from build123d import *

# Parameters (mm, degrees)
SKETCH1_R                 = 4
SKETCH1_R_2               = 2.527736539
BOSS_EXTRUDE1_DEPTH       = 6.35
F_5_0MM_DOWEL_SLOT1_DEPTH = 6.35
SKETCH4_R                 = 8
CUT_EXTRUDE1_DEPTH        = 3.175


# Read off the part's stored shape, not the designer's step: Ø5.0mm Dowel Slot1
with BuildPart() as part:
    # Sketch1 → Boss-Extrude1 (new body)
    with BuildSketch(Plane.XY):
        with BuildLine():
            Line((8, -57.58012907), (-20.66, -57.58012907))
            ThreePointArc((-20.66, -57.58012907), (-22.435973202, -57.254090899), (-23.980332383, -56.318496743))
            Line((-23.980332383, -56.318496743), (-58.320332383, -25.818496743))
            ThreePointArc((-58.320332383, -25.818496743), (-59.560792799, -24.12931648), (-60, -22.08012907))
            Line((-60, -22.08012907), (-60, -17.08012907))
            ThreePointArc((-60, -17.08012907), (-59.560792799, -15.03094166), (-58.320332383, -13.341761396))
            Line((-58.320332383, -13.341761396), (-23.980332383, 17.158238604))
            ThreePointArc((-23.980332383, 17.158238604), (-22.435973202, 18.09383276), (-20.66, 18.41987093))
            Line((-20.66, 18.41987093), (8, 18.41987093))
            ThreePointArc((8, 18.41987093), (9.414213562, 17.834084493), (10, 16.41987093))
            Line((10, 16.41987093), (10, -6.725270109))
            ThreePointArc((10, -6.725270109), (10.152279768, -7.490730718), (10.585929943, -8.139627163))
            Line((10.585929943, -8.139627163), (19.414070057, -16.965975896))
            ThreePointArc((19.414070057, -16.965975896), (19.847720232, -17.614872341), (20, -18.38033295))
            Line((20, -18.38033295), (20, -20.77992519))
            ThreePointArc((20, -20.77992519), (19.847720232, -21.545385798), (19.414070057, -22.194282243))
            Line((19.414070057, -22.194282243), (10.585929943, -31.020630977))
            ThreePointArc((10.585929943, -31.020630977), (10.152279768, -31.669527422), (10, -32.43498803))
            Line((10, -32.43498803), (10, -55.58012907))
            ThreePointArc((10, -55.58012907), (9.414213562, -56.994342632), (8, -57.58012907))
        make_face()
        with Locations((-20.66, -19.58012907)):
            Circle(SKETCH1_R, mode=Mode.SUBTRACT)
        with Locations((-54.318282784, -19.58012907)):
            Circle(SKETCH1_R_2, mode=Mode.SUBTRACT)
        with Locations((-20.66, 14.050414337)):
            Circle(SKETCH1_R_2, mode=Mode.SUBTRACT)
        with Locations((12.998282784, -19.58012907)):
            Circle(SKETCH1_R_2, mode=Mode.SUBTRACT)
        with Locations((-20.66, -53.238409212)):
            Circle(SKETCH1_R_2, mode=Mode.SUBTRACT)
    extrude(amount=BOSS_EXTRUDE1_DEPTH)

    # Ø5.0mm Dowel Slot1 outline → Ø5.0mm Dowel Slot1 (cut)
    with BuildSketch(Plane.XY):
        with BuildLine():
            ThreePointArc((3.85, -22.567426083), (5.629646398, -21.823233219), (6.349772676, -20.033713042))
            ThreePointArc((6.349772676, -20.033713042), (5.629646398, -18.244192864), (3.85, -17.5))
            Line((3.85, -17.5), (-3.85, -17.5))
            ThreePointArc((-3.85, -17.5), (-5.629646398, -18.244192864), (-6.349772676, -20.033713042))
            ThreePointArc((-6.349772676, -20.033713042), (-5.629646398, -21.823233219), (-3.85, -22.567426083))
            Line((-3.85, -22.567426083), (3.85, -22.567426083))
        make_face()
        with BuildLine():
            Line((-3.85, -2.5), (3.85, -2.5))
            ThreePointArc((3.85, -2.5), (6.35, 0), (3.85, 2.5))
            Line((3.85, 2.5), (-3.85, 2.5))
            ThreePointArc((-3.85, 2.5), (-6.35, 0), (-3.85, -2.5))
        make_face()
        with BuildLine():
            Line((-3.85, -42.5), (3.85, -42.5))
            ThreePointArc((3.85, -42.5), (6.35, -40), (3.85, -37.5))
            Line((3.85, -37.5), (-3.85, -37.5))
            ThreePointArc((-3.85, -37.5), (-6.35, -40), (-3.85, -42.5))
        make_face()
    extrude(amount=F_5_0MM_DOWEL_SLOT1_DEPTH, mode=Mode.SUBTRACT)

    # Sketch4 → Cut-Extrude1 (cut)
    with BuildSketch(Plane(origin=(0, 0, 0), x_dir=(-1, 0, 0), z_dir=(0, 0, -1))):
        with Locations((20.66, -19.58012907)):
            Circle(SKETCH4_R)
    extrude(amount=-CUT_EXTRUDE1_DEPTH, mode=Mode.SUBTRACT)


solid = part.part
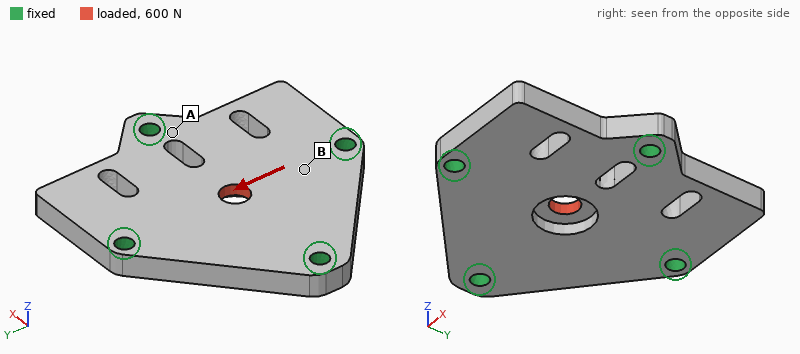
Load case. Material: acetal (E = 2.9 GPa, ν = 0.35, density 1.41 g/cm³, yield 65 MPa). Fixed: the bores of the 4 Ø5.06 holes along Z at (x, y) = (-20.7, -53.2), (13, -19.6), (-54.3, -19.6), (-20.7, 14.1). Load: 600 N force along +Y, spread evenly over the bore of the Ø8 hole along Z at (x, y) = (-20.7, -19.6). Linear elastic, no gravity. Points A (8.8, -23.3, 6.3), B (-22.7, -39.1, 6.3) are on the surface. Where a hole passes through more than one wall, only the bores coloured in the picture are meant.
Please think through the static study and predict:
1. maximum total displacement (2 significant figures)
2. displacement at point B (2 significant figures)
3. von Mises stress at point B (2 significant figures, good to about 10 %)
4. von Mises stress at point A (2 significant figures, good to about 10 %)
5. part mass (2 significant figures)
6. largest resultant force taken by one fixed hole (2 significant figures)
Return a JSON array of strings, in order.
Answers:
["38 µm", "12 µm", "3.0 MPa", "1.2 MPa", "34 g", "230 N"]
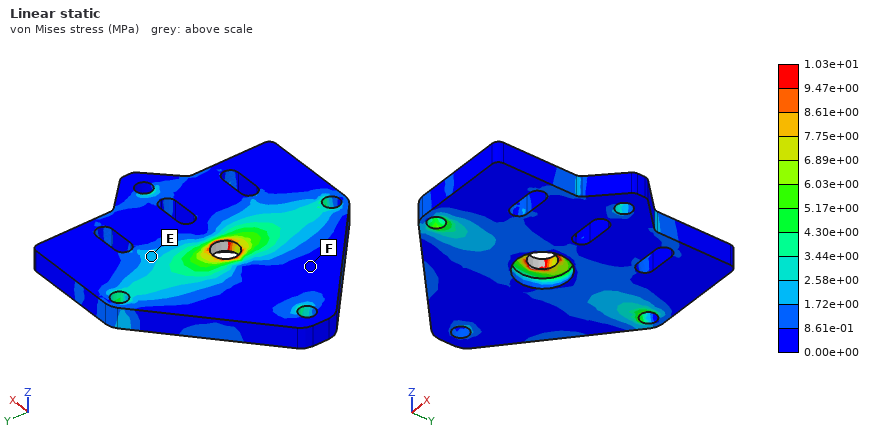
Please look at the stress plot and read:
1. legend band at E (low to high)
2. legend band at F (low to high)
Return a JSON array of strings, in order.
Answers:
["1.72e+00 to 2.58e+00 MPa", "0.00e+00 to 8.61e-01 MPa"]
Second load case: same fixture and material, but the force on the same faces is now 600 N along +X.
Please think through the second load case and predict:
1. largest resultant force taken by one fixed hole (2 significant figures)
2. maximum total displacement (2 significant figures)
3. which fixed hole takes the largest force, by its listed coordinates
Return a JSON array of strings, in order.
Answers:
["250 N", "43 µm", "(-54.3, -19.6)"]
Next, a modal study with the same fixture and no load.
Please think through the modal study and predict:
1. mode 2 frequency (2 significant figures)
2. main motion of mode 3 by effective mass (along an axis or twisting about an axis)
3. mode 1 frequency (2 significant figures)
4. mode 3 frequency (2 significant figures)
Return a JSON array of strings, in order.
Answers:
["2400 Hz", "along Z", "2400 Hz", "2700 Hz"]
